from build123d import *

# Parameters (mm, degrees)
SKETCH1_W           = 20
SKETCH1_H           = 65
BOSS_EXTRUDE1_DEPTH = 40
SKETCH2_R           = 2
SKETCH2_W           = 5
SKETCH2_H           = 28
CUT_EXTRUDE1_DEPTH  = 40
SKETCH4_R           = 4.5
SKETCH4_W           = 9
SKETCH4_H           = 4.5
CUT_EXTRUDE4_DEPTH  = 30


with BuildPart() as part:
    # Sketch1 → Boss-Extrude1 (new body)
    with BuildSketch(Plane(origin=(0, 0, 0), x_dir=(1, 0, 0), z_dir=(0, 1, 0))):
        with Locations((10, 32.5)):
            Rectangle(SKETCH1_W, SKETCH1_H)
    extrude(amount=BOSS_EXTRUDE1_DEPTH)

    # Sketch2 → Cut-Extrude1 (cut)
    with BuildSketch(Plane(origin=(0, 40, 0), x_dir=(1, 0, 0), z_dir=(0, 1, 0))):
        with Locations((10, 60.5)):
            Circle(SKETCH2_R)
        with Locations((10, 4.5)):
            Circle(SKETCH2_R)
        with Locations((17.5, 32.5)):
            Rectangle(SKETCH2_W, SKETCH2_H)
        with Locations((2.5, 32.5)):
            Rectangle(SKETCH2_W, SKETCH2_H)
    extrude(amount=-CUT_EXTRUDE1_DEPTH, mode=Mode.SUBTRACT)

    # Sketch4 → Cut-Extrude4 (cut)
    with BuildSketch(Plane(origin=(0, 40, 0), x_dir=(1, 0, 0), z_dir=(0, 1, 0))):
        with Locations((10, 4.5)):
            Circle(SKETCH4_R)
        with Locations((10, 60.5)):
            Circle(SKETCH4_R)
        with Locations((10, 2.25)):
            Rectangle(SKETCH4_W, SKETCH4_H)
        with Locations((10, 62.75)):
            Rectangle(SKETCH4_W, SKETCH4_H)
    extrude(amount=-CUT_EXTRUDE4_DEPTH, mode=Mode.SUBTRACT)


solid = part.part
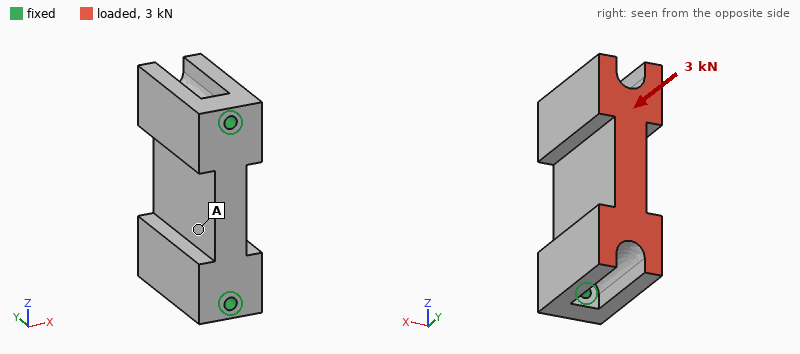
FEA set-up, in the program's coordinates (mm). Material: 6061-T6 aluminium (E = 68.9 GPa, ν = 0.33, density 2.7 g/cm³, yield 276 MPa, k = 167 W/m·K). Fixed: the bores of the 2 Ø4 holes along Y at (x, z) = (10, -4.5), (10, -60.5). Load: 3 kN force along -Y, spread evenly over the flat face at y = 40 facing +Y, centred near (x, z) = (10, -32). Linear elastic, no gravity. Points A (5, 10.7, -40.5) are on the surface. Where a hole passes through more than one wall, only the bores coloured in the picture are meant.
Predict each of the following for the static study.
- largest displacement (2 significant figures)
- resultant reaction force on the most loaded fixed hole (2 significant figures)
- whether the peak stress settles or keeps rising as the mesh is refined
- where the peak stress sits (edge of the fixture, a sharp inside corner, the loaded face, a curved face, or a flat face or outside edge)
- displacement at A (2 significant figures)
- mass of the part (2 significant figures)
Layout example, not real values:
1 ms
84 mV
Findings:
4.6 µm
1.6 kN
keeps rising
edge of the fixture
3.8 µm
98 g
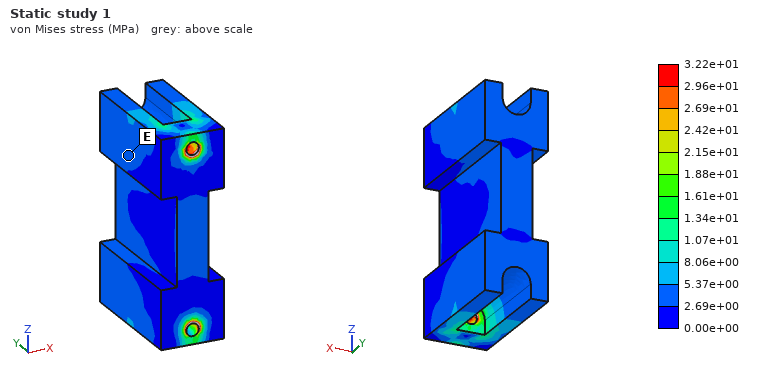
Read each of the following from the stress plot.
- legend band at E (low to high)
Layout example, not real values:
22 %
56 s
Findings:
2.69e+00 to 5.37e+00 MPa
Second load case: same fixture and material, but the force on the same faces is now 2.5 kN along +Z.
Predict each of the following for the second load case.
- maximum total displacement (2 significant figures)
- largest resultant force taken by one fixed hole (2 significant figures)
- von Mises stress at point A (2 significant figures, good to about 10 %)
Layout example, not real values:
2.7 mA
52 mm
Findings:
13 µm
2.0 kN
5.8 MPa
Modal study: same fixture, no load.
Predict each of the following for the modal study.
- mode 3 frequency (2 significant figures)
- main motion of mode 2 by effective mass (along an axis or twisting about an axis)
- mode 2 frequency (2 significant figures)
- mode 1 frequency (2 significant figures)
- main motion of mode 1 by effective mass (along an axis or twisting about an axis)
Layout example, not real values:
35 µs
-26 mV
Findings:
11 kHz
twisting about Y
8000 Hz
4600 Hz
along X
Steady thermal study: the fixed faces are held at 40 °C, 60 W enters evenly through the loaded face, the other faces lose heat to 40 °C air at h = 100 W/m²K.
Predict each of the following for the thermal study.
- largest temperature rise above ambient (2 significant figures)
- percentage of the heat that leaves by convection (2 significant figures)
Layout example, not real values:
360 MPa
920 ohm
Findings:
18 K
15 %
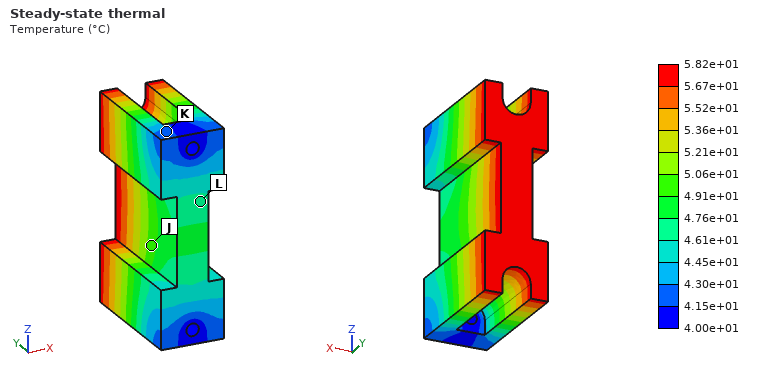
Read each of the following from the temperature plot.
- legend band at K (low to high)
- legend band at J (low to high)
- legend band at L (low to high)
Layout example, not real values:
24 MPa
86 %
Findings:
4.15e+01 to 4.30e+01 °C
4.91e+01 to 5.06e+01 °C
4.61e+01 to 4.76e+01 °C
